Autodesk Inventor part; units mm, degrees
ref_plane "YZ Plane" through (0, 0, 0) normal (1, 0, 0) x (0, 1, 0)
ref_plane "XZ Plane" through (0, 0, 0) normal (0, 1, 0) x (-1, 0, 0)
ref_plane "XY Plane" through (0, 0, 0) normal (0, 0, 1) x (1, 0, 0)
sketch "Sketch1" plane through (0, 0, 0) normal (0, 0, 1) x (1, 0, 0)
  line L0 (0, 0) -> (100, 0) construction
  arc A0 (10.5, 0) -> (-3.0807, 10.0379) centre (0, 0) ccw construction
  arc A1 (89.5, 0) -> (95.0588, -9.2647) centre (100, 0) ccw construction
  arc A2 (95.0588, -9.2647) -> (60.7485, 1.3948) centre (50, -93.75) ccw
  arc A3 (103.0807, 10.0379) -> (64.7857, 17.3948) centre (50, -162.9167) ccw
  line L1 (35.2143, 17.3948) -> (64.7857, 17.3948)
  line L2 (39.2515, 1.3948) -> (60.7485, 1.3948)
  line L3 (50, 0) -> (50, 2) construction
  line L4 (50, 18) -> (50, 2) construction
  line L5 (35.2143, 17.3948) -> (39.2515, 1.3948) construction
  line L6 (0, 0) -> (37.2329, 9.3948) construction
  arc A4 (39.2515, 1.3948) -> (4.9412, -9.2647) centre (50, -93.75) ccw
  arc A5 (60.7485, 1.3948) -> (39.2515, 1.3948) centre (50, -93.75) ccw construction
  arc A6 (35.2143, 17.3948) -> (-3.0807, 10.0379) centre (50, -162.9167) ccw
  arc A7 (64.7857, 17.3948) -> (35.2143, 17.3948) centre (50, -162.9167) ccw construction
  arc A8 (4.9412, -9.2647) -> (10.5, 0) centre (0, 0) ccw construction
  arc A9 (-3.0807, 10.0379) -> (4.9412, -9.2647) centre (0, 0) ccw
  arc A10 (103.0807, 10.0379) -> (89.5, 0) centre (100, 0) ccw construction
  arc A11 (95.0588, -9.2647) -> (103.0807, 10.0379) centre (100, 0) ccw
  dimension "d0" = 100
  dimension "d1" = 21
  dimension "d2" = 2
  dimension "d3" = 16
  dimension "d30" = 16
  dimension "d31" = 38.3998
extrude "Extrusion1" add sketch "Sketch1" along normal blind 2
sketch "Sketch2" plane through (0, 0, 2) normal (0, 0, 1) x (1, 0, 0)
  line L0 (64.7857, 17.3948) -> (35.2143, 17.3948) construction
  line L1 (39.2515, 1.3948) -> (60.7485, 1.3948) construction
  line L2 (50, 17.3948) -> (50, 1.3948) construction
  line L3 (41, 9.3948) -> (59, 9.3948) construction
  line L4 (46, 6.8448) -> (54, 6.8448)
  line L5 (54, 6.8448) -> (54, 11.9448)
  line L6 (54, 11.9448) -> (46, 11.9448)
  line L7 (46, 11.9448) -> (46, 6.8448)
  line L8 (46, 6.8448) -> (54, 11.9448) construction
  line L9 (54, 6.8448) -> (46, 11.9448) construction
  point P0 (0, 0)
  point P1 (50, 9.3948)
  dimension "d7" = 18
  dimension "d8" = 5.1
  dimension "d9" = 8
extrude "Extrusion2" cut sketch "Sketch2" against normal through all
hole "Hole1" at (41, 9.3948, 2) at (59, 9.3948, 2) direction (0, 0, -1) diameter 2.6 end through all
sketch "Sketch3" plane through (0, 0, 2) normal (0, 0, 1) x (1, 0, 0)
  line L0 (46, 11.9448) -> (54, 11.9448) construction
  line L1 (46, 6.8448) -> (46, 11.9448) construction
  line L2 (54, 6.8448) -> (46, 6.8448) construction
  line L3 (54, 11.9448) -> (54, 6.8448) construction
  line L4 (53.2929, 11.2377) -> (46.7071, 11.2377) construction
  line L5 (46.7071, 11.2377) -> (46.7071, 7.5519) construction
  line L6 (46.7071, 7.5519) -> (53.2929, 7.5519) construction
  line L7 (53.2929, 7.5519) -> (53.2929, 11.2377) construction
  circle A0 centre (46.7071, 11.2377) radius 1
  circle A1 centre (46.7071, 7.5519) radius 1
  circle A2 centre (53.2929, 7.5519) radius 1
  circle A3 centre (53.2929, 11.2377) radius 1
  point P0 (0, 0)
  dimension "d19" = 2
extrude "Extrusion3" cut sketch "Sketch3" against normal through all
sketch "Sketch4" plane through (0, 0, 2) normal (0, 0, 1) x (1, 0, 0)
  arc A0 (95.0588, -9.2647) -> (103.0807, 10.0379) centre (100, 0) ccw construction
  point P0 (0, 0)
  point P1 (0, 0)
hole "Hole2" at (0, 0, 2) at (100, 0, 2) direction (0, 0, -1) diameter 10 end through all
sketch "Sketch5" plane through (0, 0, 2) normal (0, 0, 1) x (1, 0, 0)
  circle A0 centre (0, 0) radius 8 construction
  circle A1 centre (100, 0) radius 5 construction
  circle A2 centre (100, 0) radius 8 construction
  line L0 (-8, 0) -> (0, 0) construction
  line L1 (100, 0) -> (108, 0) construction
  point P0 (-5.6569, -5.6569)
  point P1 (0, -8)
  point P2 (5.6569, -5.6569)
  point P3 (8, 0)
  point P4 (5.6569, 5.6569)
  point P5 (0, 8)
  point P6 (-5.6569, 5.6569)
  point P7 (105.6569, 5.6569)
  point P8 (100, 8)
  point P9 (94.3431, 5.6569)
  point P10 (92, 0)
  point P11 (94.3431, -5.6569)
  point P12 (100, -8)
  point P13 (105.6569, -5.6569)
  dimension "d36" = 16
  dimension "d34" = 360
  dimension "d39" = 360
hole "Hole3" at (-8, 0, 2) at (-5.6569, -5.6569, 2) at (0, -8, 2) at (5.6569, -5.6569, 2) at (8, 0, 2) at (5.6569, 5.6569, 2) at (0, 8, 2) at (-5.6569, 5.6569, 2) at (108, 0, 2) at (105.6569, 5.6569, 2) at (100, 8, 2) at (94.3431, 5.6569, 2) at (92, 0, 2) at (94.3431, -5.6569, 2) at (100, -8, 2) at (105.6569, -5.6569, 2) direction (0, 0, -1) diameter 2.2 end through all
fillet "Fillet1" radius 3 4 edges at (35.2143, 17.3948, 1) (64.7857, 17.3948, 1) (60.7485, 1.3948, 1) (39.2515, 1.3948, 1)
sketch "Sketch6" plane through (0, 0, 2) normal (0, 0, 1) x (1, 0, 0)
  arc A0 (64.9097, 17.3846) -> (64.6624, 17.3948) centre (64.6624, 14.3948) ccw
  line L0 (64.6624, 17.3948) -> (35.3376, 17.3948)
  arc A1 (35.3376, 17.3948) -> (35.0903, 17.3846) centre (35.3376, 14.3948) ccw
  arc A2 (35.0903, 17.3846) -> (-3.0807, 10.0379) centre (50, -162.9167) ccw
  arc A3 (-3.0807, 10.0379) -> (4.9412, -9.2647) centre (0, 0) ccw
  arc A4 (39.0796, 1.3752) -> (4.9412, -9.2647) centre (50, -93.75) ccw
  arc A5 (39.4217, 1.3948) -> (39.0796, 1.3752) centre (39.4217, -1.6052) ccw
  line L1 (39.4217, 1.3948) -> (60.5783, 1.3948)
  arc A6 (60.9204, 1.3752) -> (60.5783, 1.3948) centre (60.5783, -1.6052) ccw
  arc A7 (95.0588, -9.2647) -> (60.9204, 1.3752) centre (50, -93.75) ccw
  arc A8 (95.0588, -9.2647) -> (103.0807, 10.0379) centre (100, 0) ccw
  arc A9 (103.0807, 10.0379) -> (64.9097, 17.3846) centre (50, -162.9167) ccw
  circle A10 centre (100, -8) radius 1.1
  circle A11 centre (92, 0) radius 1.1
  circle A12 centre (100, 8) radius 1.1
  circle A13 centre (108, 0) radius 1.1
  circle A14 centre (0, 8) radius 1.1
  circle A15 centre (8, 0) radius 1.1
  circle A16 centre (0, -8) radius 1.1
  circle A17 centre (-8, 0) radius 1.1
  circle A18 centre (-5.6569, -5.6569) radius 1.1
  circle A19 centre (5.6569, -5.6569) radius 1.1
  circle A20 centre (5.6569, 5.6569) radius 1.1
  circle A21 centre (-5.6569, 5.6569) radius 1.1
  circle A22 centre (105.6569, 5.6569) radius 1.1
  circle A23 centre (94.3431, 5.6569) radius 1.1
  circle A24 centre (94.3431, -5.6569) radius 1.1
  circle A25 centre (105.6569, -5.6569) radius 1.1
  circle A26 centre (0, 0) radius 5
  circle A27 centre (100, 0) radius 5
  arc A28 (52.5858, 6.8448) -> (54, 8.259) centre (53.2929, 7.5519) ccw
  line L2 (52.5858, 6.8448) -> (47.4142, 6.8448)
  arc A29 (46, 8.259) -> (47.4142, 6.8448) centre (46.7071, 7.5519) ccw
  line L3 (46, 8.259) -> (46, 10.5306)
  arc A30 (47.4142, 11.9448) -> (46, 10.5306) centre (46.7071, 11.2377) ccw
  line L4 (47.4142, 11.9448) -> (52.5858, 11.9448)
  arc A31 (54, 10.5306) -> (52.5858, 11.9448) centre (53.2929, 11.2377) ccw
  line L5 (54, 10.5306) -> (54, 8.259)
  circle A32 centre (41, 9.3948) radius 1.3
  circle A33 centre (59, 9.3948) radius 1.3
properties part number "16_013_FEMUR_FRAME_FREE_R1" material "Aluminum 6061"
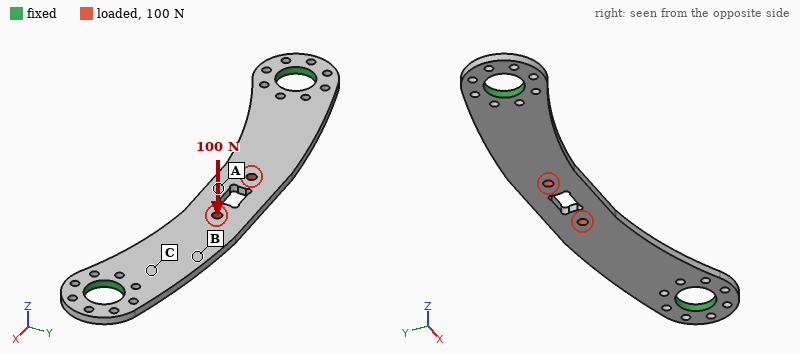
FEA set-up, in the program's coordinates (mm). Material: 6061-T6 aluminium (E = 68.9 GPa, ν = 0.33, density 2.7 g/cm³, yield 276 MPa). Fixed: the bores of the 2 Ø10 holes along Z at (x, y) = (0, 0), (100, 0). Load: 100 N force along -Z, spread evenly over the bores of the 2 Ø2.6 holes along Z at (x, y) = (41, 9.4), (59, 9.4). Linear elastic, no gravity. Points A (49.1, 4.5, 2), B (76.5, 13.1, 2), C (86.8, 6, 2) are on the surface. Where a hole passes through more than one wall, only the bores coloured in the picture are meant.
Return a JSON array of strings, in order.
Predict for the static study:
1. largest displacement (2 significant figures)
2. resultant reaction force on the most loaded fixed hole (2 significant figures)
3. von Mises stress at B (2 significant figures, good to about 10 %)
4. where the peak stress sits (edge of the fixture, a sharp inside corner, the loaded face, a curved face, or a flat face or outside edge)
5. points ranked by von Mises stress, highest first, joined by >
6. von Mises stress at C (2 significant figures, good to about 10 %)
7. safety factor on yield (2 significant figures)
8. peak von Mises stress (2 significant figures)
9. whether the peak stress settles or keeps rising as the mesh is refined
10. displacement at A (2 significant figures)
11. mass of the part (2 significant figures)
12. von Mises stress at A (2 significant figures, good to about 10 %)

["0.64 mm", "50 N", "19 MPa", "a curved face", "A > C > B", "51 MPa", "1.3", "210 MPa", "settles", "0.55 mm", "10 g", "95 MPa"]
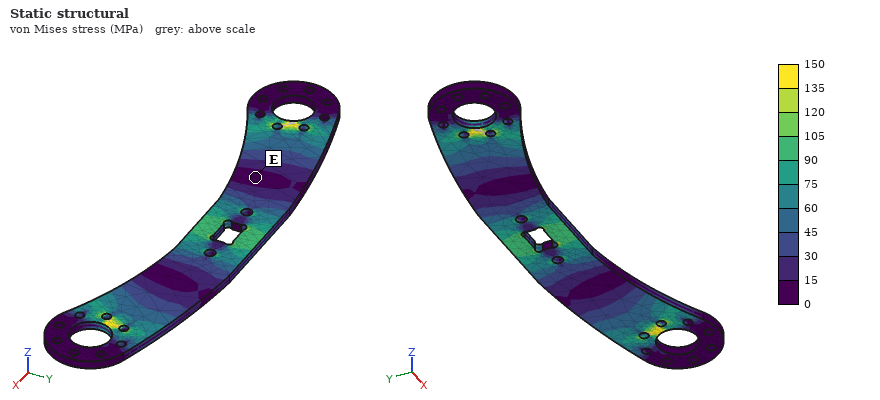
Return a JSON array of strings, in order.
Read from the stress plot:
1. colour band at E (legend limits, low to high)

["0 to 15 MPa"]
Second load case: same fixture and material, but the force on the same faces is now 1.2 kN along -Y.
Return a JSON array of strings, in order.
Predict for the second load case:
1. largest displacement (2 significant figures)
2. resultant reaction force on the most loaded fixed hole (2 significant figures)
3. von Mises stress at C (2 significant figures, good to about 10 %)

["0.11 mm", "960 N", "29 MPa"]
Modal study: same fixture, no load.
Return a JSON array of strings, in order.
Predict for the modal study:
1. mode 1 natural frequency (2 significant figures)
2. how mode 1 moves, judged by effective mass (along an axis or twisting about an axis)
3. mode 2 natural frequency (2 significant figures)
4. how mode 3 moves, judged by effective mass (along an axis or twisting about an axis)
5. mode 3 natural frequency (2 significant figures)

["1200 Hz", "along Z", "3100 Hz", "twisting about X", "4200 Hz"]
